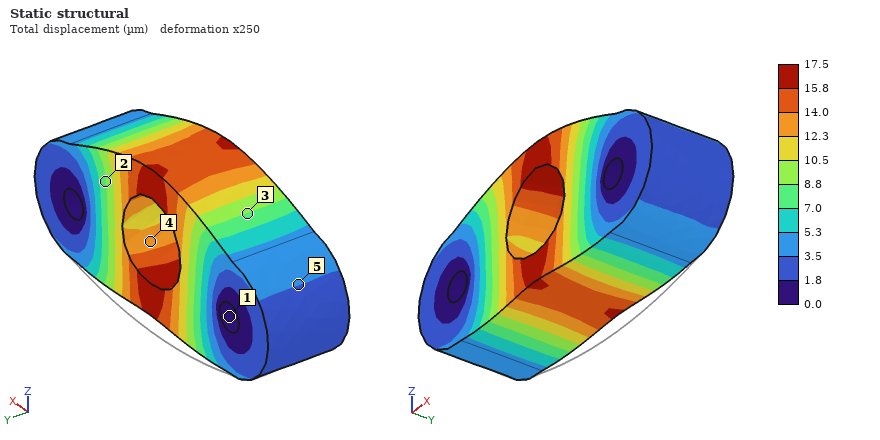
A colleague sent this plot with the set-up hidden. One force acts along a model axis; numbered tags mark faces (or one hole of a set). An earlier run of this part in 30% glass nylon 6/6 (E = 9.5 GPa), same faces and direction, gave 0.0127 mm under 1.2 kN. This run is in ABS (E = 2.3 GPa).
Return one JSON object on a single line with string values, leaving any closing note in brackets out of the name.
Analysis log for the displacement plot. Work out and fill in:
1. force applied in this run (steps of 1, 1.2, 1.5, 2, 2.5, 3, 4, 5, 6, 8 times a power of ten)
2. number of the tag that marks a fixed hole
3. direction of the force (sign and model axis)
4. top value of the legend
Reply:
{"force applied in this run": "400 N", "number of the tag that marks a fixed hole": "1", "direction of the force": "+Z", "top value of the legend": "17.5 µm"}
